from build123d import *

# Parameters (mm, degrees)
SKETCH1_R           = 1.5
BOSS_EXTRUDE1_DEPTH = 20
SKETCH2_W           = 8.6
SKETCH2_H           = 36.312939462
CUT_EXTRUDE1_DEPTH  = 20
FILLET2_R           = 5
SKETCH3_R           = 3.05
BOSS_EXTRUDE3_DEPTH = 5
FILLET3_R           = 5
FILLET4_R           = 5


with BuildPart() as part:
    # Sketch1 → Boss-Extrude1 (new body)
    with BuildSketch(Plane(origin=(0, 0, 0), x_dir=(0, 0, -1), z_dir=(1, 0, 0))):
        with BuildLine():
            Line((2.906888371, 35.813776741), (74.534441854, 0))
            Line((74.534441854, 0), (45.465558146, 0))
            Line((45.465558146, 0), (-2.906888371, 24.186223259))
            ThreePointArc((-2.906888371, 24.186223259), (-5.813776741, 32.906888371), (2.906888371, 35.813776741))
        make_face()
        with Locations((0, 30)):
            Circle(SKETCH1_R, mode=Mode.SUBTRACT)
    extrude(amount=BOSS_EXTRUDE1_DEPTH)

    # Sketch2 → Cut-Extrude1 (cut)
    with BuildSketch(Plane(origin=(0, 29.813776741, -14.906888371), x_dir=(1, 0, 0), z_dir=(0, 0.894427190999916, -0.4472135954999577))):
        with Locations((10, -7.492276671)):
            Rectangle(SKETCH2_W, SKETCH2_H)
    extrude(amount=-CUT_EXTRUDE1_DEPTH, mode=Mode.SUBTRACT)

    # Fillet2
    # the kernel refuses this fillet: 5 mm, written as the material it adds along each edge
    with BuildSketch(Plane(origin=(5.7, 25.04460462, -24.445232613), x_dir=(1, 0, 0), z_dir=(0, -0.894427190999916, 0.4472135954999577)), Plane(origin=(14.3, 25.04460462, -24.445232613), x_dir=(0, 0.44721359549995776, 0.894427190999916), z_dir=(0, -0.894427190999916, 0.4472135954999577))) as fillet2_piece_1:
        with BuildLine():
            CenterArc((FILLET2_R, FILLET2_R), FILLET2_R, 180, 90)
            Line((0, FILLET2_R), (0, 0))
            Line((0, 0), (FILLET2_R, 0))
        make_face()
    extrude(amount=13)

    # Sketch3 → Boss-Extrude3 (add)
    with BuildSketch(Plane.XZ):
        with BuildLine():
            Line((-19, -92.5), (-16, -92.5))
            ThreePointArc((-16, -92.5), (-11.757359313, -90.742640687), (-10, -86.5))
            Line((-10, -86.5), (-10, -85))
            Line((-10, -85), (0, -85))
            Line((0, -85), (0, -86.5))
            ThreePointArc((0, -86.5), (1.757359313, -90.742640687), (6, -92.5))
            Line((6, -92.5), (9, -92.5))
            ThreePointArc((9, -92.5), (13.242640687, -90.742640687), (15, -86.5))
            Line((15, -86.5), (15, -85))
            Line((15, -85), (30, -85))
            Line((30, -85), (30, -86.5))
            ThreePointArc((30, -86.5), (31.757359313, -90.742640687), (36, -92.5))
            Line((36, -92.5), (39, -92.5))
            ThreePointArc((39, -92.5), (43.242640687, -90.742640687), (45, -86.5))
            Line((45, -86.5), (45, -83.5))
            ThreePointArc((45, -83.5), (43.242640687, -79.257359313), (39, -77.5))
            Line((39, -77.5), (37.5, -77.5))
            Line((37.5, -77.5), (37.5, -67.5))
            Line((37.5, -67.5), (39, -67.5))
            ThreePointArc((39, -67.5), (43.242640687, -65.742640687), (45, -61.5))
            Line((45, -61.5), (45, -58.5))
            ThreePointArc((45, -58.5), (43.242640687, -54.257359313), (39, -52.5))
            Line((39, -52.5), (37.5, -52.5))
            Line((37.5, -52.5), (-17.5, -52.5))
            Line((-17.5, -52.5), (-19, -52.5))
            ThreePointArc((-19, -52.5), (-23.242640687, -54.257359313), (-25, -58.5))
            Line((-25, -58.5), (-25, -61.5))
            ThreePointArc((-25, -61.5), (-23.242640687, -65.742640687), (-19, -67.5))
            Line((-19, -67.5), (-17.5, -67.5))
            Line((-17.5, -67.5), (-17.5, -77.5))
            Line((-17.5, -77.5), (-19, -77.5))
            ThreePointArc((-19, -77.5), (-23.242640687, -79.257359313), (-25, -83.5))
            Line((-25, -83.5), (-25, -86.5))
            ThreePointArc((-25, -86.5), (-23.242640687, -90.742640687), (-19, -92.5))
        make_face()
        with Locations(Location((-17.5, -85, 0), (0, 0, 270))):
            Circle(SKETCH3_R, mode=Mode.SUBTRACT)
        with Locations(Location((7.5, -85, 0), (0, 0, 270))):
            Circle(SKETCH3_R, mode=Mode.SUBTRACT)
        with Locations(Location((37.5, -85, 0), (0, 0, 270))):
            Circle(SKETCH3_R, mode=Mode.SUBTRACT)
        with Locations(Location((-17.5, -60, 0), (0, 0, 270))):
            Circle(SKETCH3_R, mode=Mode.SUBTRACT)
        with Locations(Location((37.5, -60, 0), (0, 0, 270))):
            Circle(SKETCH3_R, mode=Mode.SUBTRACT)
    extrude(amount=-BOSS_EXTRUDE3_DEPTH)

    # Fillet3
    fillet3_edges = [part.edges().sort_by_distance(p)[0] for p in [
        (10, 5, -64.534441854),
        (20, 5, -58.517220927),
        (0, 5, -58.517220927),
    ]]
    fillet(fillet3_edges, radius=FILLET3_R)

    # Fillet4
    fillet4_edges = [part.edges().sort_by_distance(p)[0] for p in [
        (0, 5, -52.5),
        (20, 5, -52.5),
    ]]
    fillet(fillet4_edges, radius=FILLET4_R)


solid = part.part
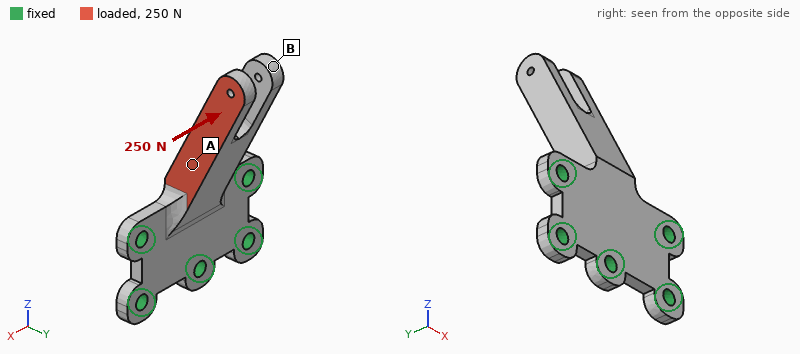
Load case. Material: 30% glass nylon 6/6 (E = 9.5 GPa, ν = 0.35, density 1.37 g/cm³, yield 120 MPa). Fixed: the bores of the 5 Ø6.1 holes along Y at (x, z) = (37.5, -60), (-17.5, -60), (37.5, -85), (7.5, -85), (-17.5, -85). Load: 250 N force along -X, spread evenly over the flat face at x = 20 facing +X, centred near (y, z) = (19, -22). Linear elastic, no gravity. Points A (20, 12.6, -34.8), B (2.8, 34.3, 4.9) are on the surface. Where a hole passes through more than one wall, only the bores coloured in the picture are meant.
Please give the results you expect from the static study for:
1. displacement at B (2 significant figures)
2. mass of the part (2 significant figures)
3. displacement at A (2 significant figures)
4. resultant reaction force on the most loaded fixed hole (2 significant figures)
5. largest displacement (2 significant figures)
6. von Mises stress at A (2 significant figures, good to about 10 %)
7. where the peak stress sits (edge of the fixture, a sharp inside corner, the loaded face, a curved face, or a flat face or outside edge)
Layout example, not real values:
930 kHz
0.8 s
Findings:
0.22 mm
34 g
0.072 mm
190 N
0.47 mm
5.2 MPa
a curved face
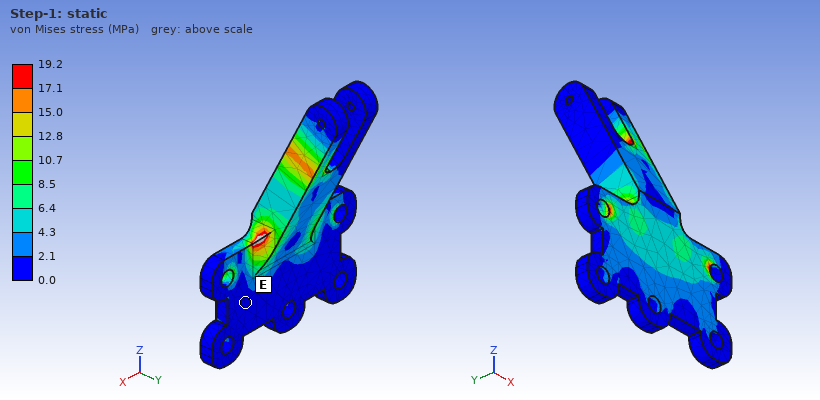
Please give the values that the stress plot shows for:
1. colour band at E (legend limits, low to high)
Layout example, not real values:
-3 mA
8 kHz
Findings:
0.0 to 2.1 MPa
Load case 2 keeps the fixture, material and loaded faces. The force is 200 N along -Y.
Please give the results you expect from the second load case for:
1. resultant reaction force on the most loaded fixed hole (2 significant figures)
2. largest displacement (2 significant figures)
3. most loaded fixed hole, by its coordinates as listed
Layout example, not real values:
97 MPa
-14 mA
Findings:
310 N
1.5 mm
(37.5, -60)
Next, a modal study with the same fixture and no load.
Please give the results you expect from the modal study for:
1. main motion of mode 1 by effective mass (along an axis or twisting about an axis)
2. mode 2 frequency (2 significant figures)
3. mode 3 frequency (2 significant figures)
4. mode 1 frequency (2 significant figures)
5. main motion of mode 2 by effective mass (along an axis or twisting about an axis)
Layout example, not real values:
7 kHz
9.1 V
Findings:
along Y
1600 Hz
2700 Hz
600 Hz
along X
